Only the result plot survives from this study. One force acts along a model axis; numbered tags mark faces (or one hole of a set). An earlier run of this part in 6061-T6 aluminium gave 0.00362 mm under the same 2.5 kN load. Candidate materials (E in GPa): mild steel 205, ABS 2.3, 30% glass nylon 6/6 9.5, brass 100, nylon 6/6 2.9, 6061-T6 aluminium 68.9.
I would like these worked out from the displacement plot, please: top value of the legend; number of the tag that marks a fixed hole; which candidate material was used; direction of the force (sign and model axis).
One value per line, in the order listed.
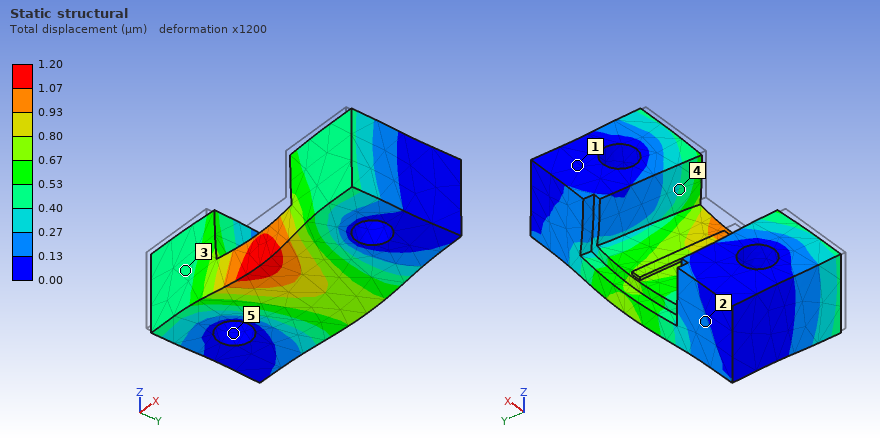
1.20 µm
5
mild steel
+Y
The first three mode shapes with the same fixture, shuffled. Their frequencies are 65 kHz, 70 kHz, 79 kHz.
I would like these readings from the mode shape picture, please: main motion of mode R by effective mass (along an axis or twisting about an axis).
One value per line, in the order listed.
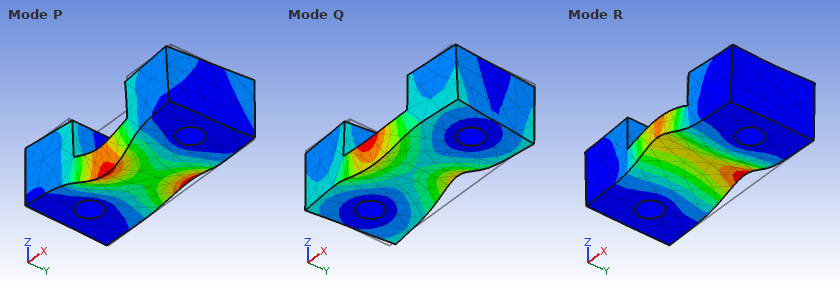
along Z
